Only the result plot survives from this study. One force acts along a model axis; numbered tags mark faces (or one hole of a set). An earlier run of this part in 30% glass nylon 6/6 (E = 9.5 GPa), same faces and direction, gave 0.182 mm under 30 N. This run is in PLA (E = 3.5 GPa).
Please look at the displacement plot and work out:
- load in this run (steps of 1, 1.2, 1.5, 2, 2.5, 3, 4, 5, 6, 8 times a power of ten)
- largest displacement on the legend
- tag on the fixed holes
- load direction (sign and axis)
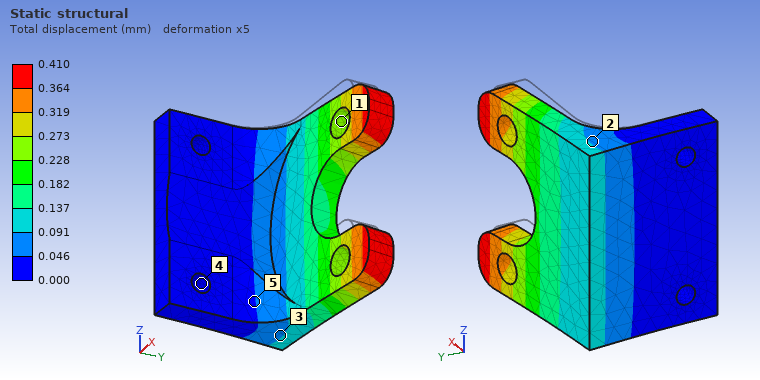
25 N
0.410 mm
4
+Y
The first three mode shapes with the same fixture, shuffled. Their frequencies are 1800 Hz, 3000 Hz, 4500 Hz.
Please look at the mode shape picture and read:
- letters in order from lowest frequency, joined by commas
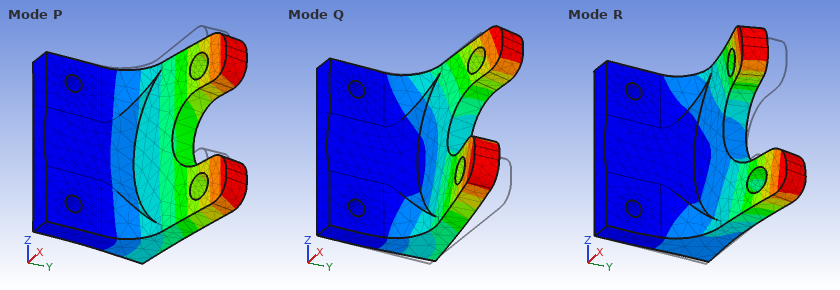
P, Q, R
